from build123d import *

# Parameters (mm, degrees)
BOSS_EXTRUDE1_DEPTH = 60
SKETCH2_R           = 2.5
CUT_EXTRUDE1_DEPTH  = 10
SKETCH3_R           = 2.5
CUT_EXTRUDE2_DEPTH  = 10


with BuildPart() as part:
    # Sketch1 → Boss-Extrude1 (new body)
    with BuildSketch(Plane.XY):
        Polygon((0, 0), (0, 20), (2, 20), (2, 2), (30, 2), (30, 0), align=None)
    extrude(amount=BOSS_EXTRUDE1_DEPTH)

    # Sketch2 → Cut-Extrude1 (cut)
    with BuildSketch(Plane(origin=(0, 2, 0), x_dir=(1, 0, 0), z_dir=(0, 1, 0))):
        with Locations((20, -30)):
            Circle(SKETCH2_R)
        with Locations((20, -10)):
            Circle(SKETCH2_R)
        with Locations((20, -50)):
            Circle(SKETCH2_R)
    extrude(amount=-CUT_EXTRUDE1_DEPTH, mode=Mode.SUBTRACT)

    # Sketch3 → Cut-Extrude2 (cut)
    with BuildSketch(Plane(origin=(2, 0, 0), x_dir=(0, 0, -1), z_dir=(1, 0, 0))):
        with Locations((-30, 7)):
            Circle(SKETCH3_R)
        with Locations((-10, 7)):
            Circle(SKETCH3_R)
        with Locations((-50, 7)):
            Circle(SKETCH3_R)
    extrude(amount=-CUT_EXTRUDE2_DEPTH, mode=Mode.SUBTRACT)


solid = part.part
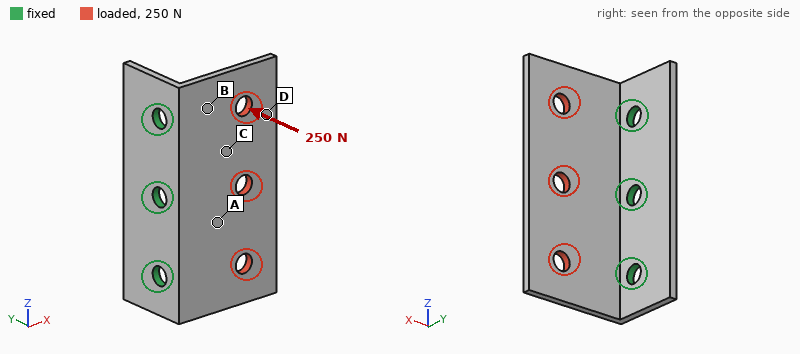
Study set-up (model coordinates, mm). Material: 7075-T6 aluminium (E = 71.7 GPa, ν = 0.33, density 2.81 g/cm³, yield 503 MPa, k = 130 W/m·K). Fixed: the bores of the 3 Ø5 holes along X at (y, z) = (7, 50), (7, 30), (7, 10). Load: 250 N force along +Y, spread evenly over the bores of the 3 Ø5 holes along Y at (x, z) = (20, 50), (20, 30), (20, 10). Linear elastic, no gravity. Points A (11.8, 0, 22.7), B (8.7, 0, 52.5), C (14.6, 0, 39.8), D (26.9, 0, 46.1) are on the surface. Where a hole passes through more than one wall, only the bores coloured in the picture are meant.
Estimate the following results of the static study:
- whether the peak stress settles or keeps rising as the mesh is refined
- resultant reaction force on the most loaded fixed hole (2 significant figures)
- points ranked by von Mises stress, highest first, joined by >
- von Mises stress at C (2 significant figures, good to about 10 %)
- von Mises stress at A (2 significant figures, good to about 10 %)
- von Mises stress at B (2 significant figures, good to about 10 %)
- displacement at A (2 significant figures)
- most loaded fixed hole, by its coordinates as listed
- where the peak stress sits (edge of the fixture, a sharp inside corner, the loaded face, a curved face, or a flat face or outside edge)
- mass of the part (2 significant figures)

keeps rising
100 N
B > A > C > D
30 MPa
45 MPa
64 MPa
0.15 mm
(7, 30)
edge of the fixture
16 g
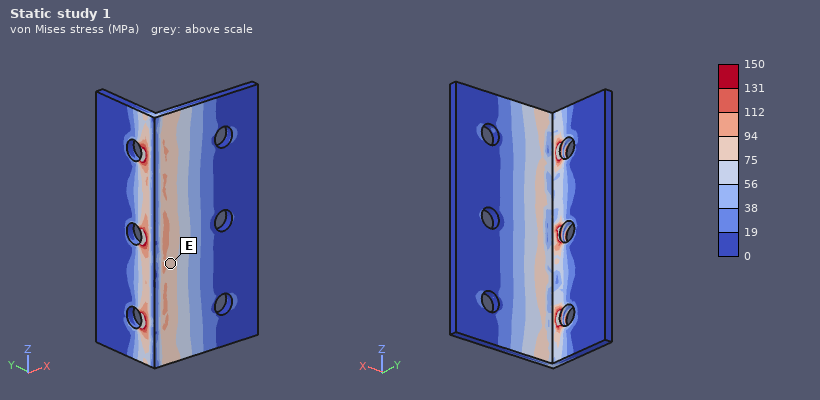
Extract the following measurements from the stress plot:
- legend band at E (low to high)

75 to 94 MPa
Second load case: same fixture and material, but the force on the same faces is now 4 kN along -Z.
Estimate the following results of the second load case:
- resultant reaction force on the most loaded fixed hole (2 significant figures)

2.2 kN
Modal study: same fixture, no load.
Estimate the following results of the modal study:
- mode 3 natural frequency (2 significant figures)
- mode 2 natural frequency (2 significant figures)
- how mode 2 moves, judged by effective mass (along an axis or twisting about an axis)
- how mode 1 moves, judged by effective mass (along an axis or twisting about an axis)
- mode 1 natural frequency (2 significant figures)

5200 Hz
2600 Hz
twisting about X
along Y
1600 Hz
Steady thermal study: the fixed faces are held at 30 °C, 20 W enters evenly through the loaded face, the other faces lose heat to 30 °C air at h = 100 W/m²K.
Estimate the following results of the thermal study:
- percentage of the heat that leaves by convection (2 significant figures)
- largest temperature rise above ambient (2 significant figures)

32 %
27 K
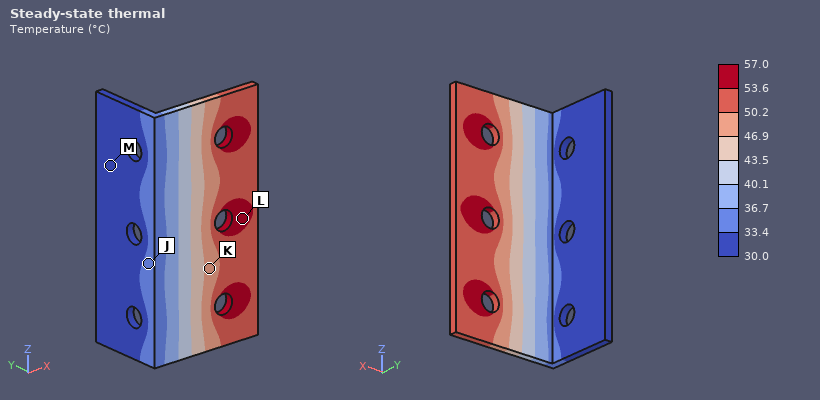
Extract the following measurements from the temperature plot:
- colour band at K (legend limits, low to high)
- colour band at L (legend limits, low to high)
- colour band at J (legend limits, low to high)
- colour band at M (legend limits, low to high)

46.9 to 50.2 °C
53.6 to 57.0 °C
33.4 to 36.7 °C
30.0 to 33.4 °C
